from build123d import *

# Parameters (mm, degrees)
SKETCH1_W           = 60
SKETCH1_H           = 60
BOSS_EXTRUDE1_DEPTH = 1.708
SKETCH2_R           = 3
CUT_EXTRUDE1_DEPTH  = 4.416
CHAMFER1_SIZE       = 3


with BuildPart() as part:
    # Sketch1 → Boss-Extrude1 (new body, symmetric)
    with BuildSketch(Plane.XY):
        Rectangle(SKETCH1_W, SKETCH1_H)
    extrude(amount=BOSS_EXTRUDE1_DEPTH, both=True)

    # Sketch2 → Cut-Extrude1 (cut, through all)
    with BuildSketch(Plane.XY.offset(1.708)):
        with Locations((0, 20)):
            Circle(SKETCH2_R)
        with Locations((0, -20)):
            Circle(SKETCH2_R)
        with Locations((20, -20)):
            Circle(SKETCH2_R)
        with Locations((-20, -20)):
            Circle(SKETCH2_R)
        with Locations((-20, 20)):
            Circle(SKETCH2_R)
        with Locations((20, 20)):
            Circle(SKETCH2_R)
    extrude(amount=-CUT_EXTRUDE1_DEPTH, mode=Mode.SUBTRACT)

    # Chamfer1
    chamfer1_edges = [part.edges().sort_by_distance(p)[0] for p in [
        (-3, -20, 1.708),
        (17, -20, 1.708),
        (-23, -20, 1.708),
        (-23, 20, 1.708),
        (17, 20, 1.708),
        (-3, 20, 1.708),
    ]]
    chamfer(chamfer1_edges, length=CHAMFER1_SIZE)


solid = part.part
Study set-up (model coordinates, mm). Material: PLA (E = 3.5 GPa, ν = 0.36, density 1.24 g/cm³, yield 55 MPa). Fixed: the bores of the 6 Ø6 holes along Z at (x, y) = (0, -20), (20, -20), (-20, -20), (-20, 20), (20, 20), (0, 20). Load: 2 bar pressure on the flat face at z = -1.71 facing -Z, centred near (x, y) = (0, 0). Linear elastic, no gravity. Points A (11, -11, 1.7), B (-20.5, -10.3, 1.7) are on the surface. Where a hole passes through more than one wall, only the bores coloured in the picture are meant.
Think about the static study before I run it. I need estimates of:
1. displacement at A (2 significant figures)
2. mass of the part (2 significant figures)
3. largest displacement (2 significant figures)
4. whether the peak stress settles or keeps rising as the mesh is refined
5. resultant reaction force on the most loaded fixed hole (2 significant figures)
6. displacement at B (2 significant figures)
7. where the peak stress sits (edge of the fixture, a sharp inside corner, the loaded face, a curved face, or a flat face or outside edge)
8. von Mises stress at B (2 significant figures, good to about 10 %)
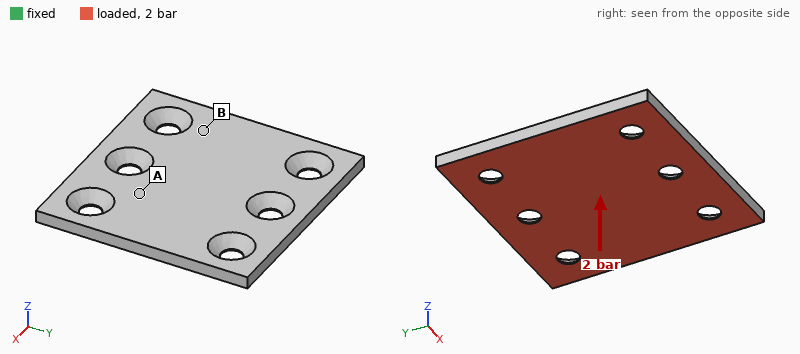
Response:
0.087 mm
14 g
0.21 mm
keeps rising
150 N
0.10 mm
edge of the fixture
7.3 MPa
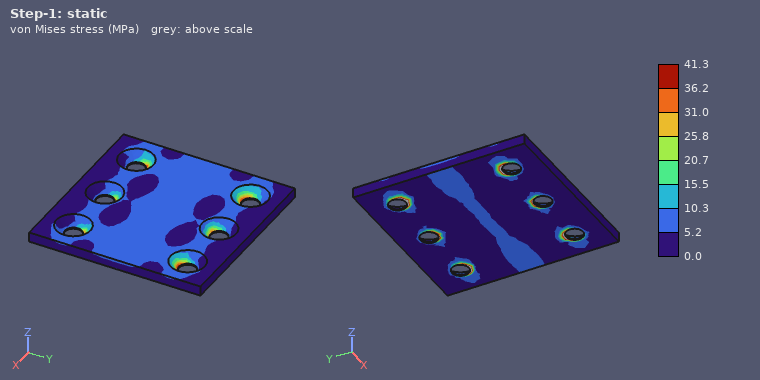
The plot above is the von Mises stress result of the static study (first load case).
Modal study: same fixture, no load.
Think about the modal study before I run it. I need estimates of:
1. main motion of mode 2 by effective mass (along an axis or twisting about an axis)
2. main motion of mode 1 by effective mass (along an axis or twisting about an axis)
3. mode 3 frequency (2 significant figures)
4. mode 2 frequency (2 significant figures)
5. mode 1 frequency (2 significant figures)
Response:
twisting about Y
along Z
4100 Hz
3000 Hz
2800 Hz
